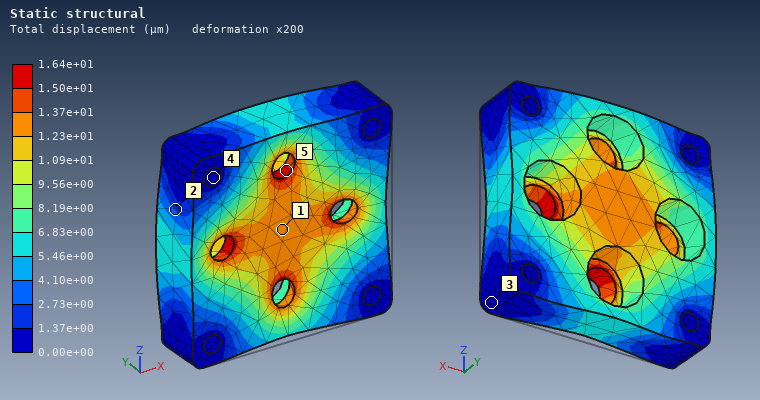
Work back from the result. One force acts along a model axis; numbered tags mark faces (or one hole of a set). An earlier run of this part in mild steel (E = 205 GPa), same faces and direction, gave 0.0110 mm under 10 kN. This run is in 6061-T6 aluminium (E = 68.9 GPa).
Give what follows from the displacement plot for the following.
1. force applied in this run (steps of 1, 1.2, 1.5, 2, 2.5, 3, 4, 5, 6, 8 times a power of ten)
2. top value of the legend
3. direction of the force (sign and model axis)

5 kN
1.64e+01 µm
+Y
